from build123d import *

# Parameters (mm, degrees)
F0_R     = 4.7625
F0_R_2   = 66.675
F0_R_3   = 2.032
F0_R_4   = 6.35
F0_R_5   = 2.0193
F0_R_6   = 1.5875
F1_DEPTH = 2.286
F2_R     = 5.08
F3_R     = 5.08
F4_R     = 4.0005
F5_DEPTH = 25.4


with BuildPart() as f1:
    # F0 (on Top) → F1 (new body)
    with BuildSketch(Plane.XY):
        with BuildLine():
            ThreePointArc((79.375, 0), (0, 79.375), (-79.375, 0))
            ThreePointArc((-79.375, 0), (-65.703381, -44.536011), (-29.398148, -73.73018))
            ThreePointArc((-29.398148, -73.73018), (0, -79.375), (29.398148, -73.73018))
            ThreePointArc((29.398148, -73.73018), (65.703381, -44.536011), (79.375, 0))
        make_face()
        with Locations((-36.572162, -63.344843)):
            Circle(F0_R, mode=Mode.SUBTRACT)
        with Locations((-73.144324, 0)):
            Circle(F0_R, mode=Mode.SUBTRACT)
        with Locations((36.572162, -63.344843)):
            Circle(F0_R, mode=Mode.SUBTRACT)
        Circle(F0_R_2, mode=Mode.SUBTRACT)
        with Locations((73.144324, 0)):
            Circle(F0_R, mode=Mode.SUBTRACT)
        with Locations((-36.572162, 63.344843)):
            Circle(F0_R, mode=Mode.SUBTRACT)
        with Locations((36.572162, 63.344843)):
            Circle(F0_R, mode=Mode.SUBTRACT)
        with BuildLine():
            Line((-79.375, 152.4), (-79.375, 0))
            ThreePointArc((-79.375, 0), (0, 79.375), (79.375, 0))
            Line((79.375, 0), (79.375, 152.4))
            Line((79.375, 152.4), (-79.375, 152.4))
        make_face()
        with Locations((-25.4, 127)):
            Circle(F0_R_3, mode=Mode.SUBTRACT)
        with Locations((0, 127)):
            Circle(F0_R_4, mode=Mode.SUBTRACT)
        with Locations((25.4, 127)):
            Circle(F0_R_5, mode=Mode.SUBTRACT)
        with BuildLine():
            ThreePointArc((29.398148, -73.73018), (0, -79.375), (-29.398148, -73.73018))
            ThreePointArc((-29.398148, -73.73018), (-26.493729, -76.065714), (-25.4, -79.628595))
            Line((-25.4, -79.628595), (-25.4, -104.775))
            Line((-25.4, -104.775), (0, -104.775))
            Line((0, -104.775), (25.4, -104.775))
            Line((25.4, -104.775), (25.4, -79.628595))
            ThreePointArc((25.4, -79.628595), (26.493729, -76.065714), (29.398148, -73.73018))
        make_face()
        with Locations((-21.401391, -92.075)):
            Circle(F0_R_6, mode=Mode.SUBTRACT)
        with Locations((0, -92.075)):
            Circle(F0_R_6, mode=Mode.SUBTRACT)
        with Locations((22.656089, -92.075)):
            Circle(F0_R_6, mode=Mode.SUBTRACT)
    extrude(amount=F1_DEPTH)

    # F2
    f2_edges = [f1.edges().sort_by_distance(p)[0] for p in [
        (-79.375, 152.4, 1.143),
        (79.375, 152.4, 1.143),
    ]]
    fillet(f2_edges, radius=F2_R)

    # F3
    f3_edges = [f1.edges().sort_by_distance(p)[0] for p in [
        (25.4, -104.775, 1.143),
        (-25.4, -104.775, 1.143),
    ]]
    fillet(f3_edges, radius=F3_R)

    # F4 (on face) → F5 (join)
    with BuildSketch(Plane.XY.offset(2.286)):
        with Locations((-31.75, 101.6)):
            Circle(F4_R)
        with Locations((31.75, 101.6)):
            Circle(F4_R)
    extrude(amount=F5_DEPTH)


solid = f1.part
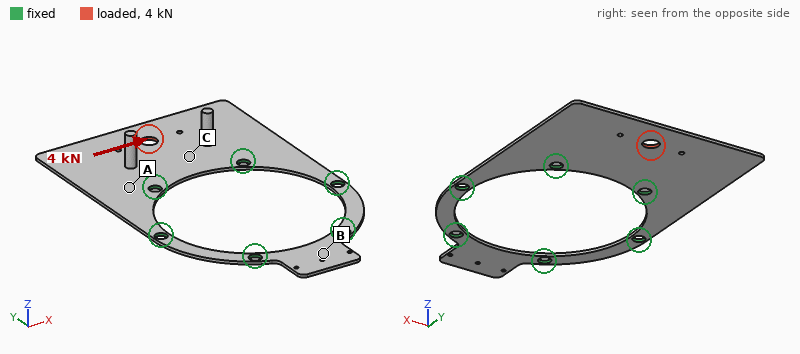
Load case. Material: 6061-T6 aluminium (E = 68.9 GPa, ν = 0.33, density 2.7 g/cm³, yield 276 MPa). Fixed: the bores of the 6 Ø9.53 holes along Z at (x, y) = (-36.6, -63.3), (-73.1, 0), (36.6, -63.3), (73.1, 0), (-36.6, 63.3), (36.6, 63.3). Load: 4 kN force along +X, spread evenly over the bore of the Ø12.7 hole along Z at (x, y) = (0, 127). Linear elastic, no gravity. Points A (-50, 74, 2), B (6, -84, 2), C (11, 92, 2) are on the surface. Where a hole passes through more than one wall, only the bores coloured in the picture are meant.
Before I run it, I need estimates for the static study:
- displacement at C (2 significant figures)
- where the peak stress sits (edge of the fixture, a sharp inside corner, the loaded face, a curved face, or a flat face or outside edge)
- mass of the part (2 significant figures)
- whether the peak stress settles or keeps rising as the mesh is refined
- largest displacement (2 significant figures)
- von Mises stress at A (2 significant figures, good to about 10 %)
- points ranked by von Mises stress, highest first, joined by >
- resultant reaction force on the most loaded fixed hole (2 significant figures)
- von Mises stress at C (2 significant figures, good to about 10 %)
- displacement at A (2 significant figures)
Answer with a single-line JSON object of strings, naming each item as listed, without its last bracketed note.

{"displacement at C": "25 µm", "where the peak stress sits": "edge of the fixture", "mass of the part": "140 g", "whether the peak stress settles or keeps rising as the mesh is refined": "keeps rising", "largest displacement": "75 µm", "von Mises stress at A": "18 MPa", "points ranked by von Mises stress, highest first, joined by >": "C > A > B", "resultant reaction force on the most loaded fixed hole": "2.6 kN", "von Mises stress at C": "33 MPa", "displacement at A": "16 µm"}
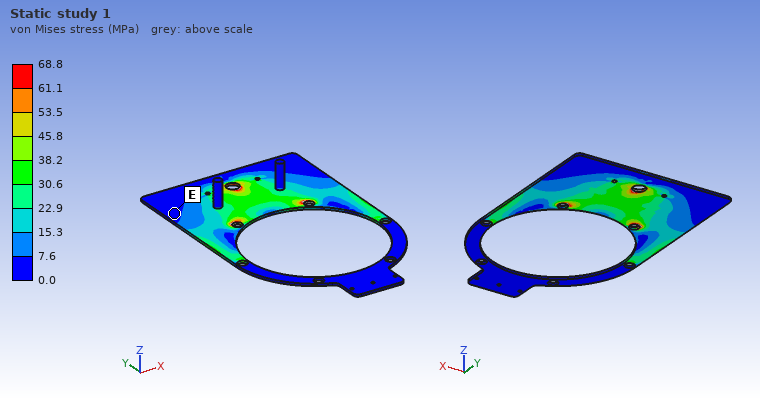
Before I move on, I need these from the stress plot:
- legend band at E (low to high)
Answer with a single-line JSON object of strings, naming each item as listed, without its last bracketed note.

{"legend band at E": "0.0 to 7.6 MPa"}
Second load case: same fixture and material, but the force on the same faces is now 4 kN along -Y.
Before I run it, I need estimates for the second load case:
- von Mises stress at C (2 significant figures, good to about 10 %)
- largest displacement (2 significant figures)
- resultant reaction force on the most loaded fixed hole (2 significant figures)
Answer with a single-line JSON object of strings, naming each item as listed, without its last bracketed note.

{"von Mises stress at C": "20 MPa", "largest displacement": "39 µm", "resultant reaction force on the most loaded fixed hole": "2.0 kN"}
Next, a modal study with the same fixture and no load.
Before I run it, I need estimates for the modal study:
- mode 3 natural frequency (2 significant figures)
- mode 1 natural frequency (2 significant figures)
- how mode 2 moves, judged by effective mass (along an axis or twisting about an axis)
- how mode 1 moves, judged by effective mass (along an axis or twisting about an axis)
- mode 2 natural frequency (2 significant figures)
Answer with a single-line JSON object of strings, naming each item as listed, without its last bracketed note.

{"mode 3 natural frequency": "660 Hz", "mode 1 natural frequency": "220 Hz", "how mode 2 moves, judged by effective mass": "twisting about Y", "how mode 1 moves, judged by effective mass": "along Z", "mode 2 natural frequency": "350 Hz"}
